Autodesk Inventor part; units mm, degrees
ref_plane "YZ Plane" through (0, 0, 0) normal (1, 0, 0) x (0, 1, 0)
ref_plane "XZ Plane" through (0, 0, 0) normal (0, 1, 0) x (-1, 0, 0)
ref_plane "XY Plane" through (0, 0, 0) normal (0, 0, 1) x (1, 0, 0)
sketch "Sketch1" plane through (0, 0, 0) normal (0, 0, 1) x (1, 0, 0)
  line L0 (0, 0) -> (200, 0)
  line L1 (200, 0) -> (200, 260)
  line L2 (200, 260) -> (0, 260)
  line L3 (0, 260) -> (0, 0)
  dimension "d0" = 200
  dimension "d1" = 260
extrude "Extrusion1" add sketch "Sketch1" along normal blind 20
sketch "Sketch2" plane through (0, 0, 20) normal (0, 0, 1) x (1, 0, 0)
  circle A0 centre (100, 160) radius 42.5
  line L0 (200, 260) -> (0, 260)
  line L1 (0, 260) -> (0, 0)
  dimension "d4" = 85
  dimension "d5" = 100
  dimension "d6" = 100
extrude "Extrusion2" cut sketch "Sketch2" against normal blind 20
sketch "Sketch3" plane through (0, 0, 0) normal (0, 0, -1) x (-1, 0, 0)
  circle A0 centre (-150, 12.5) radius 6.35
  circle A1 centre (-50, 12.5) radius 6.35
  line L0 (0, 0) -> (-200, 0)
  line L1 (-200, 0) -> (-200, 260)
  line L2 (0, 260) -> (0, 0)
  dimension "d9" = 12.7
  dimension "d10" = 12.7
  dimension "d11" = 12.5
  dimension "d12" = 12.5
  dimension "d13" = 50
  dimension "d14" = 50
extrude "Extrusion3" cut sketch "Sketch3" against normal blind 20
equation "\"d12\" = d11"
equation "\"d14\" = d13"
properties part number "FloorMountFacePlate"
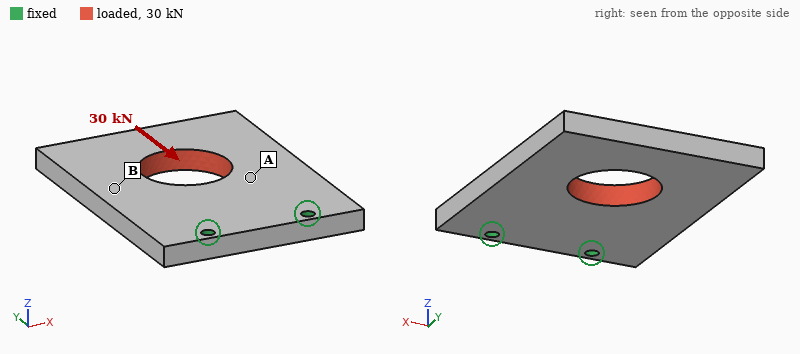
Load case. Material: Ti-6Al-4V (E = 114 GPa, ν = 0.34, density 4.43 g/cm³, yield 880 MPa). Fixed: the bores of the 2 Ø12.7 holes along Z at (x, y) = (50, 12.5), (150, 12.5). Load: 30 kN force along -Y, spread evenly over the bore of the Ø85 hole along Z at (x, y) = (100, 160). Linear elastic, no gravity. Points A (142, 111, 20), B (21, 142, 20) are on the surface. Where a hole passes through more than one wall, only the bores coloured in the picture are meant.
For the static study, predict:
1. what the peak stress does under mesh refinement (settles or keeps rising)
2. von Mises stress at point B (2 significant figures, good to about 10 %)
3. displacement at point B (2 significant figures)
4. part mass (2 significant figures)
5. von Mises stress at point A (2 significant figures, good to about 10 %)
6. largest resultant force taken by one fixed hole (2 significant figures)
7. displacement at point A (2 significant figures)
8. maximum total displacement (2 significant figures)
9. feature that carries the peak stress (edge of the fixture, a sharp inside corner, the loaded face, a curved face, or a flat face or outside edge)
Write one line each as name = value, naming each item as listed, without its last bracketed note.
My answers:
what the peak stress does under mesh refinement = keeps rising
von Mises stress at point B = 6.0 MPa
displacement at point B = 14 µm
part mass = 4.1 kg
von Mises stress at point A = 12 MPa
largest resultant force taken by one fixed hole = 15 kN
displacement at point A = 11 µm
maximum total displacement = 24 µm
feature that carries the peak stress = edge of the fixture
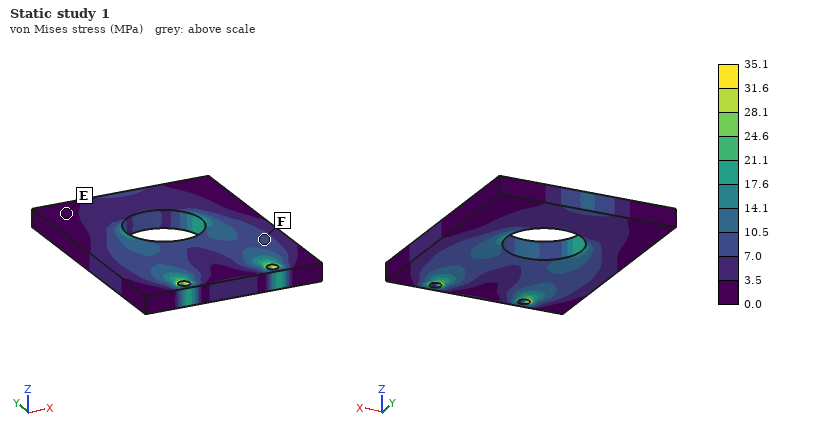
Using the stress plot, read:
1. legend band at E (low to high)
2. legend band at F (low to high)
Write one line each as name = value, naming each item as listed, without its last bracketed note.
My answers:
legend band at E = 0.0 to 3.5 MPa
legend band at F = 7.0 to 10.5 MPa
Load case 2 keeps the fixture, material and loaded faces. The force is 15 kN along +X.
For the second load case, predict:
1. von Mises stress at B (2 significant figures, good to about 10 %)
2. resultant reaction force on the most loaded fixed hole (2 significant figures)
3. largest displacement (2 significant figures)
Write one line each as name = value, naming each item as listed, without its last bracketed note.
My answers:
von Mises stress at B = 7.5 MPa
resultant reaction force on the most loaded fixed hole = 22 kN
largest displacement = 94 µm
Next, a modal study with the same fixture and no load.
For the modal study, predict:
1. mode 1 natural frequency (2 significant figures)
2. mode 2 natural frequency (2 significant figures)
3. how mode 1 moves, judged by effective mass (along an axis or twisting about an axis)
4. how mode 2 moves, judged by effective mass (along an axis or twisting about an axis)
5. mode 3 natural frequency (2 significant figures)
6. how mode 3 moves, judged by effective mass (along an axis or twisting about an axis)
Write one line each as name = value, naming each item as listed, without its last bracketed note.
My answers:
mode 1 natural frequency = 250 Hz
mode 2 natural frequency = 650 Hz
how mode 1 moves, judged by effective mass = along Z
how mode 2 moves, judged by effective mass = twisting about Y
mode 3 natural frequency = 1300 Hz
how mode 3 moves, judged by effective mass = along X
